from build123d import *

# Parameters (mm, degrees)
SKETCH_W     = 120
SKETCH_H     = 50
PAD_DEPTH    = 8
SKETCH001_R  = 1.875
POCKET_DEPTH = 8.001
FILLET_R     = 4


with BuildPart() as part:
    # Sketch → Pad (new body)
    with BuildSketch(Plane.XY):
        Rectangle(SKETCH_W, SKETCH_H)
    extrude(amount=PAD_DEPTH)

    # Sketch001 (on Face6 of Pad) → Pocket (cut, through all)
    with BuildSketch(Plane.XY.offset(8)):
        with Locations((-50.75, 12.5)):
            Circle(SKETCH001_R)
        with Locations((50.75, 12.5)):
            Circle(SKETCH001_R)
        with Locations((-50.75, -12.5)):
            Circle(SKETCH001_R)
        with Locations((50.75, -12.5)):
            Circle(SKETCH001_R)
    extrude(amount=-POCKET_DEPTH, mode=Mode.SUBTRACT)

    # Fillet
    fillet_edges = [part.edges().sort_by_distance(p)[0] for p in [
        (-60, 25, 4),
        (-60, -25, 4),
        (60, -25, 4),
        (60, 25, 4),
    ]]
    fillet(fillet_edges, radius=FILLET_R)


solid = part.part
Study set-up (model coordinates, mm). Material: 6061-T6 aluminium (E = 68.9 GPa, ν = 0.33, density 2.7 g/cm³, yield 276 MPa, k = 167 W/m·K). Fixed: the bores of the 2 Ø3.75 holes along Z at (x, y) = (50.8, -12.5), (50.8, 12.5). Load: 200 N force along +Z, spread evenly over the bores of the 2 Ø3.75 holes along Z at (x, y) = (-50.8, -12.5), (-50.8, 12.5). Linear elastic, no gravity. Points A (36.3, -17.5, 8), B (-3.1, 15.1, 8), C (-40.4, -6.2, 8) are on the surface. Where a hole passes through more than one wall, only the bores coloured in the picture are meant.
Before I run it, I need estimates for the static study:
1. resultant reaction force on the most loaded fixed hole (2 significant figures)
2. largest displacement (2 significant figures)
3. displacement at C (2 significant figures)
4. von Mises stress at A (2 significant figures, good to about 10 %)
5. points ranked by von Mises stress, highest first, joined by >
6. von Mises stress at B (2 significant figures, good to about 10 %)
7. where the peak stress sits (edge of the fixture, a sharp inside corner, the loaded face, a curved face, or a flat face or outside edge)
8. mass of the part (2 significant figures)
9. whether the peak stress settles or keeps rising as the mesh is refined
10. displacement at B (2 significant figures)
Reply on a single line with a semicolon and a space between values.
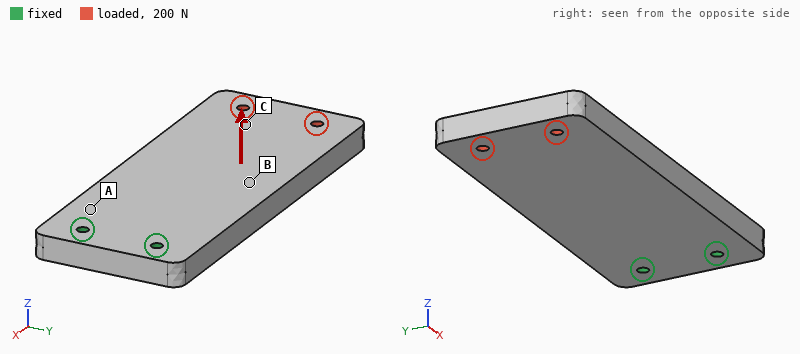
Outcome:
100 N; 0.57 mm; 0.43 mm; 32 MPa; A > B > C; 18 MPa; edge of the fixture; 130 g; keeps rising; 0.18 mm
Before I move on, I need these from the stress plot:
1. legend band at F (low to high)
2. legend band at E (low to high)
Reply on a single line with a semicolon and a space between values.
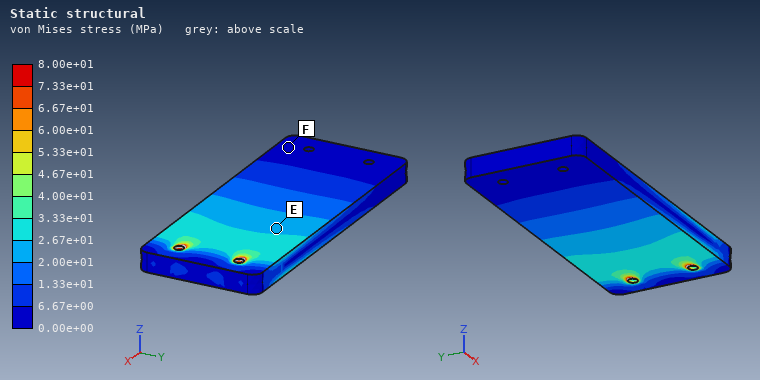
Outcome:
0.00e+00 to 6.67e+00 MPa; 2.00e+01 to 2.67e+01 MPa
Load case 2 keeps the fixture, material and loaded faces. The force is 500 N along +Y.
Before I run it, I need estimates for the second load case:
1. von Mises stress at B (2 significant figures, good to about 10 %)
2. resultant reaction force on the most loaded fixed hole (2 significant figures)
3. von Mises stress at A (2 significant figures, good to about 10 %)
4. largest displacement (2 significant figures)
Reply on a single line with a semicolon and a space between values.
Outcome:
4.8 MPa; 1.9 kN; 10 MPa; 56 µm
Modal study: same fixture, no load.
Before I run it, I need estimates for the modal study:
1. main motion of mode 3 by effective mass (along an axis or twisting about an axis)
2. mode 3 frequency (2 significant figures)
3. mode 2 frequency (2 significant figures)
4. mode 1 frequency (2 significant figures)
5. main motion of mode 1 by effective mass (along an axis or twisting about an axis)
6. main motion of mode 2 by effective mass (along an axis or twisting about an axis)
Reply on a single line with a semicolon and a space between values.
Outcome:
along Y; 2400 Hz; 2300 Hz; 520 Hz; along Z; twisting about X
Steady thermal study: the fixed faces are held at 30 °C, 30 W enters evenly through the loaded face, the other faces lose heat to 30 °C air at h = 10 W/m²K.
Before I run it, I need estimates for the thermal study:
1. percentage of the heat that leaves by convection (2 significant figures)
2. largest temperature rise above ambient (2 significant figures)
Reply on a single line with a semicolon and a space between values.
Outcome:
11 %; 46 K
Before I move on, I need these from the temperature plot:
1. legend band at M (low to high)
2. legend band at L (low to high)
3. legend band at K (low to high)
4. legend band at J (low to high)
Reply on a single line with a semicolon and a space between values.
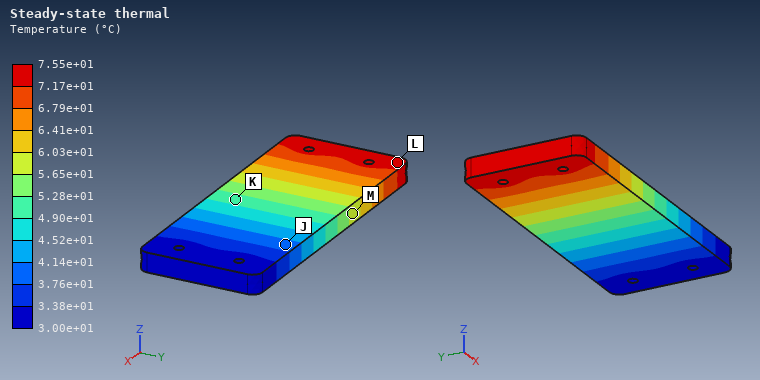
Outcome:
5.65e+01 to 6.03e+01 °C; 7.17e+01 to 7.55e+01 °C; 4.90e+01 to 5.28e+01 °C; 3.76e+01 to 4.14e+01 °C
